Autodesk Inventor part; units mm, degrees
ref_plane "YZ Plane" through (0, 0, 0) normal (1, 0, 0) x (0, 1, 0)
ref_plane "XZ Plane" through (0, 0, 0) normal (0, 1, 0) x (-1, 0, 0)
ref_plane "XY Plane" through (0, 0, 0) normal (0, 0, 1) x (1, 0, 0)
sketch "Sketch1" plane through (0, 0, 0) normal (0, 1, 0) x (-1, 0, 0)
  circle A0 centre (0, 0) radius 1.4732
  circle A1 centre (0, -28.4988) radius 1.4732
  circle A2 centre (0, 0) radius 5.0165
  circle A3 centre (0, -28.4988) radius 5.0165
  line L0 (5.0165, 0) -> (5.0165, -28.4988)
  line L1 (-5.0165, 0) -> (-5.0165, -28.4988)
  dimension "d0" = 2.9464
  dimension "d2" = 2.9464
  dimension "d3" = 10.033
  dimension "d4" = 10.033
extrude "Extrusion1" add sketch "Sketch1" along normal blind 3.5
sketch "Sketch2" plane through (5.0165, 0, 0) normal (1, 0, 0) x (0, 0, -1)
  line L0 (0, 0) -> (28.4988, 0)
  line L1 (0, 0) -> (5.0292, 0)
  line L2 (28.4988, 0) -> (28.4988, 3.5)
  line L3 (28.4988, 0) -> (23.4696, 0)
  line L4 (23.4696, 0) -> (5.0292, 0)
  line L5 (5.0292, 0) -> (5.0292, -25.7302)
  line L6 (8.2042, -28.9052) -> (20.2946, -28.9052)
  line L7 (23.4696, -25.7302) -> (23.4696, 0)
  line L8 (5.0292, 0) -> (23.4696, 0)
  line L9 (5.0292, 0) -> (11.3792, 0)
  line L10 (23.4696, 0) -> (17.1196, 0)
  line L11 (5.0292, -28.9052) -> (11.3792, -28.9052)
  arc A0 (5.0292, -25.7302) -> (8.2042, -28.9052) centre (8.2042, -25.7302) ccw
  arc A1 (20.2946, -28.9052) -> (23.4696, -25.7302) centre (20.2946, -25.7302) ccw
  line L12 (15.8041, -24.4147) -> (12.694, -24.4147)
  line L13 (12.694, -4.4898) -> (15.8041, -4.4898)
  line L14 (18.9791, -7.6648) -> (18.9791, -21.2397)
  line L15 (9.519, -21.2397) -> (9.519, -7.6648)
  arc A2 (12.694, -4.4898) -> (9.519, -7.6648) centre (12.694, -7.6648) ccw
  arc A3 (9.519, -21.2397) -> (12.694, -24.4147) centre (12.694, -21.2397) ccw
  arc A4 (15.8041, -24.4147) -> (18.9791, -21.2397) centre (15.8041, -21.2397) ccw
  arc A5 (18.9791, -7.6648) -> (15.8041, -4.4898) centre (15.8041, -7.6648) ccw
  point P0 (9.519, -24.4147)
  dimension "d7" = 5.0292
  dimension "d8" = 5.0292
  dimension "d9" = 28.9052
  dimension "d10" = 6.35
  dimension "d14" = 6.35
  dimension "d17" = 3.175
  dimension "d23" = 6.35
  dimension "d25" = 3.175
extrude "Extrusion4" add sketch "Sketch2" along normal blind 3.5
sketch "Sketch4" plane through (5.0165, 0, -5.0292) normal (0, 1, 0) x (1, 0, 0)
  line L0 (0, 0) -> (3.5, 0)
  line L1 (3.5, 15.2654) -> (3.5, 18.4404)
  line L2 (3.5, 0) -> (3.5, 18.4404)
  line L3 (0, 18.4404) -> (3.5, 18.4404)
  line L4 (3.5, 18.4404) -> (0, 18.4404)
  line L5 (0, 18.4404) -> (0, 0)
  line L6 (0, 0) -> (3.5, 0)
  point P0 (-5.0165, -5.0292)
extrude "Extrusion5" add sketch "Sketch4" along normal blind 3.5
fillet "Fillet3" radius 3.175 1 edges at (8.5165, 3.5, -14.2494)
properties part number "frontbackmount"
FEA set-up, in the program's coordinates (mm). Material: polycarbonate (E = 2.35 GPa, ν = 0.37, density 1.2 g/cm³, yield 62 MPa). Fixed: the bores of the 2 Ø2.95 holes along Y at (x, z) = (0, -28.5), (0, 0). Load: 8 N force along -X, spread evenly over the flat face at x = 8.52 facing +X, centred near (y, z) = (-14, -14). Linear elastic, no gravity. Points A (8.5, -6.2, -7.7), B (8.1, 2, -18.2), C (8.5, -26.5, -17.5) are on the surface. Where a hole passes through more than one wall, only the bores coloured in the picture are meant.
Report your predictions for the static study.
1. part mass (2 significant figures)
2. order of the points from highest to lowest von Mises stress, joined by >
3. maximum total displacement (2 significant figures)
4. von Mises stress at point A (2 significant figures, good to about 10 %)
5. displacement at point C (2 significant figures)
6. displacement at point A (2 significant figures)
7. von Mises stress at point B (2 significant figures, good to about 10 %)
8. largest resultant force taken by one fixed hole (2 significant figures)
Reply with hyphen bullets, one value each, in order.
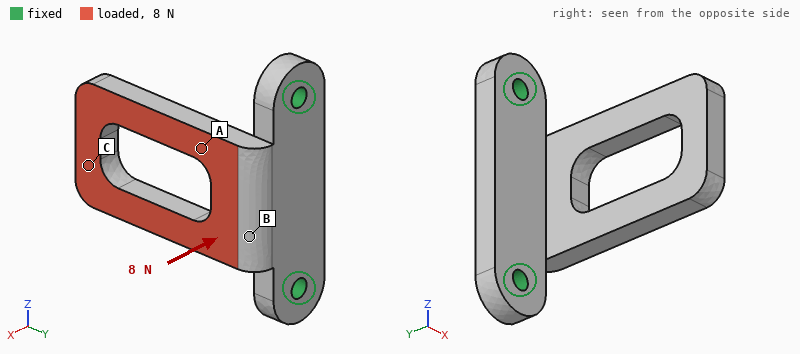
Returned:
- 3.2 g
- A > B > C
- 0.52 mm
- 3.5 MPa
- 0.47 mm
- 0.100 mm
- 1.4 MPa
- 4.3 N
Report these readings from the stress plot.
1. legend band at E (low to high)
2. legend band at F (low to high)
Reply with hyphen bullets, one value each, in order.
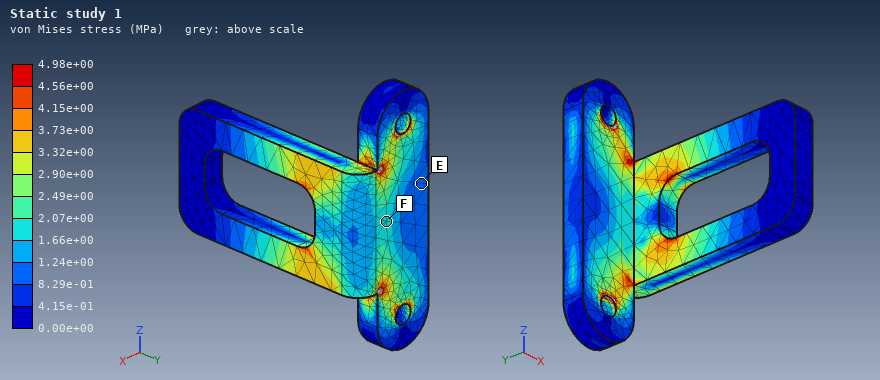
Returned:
- 8.29e-01 to 1.24e+00 MPa
- 1.66e+00 to 2.07e+00 MPa
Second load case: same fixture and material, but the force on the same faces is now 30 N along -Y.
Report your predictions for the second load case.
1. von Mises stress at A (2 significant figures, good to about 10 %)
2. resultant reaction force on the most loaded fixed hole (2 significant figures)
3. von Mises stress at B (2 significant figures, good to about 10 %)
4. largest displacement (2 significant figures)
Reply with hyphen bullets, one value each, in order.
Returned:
- 2.4 MPa
- 15 N
- 1.2 MPa
- 0.52 mm
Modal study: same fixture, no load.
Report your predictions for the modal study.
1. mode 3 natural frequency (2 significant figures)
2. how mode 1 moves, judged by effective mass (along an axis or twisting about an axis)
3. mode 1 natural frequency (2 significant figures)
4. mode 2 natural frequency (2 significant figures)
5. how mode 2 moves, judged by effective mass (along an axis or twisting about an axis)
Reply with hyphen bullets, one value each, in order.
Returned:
- 2100 Hz
- along X
- 610 Hz
- 1500 Hz
- along Z
